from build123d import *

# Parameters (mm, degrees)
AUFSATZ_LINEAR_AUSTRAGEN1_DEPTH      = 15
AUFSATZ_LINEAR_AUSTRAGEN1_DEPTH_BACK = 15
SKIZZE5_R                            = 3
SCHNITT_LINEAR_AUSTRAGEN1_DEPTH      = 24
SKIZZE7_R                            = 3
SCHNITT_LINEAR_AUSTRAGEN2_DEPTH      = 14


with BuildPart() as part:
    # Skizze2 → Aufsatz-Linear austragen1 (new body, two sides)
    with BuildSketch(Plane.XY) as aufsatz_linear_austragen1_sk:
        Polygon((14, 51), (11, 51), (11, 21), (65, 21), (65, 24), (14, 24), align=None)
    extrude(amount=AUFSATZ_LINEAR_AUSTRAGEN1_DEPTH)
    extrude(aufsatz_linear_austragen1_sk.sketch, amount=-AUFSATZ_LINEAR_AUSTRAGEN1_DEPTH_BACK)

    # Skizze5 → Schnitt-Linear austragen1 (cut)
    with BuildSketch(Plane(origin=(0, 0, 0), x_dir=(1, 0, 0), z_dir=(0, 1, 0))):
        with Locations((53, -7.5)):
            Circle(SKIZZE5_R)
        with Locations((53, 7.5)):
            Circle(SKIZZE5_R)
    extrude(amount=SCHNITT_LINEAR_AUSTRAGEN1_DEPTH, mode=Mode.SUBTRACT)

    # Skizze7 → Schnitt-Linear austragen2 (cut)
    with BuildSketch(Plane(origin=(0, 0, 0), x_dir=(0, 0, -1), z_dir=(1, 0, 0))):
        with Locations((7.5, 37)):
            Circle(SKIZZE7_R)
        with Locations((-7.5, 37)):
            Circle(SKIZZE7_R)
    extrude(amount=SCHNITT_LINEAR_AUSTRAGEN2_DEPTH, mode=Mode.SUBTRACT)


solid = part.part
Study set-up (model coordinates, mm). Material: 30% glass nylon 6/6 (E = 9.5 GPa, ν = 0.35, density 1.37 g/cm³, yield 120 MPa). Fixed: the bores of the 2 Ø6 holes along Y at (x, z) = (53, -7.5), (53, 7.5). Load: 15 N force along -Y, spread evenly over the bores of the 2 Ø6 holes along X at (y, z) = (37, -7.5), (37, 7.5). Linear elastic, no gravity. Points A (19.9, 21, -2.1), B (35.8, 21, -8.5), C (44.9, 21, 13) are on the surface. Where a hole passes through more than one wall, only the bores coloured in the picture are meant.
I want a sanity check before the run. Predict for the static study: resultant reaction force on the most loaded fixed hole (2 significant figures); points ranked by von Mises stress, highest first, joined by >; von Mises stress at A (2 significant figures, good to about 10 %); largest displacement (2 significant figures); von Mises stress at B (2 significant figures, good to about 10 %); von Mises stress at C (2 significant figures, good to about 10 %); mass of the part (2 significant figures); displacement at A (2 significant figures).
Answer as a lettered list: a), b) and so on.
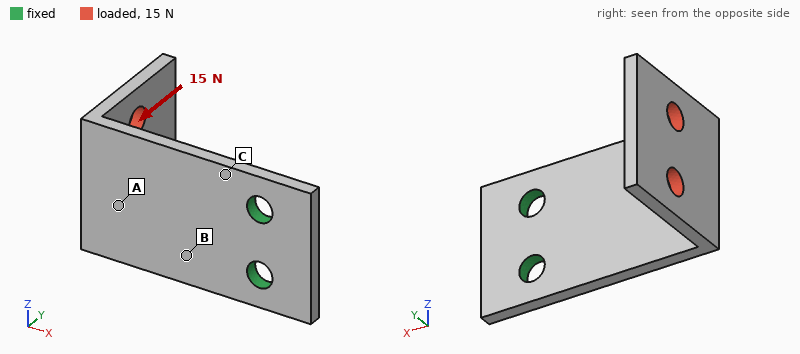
a) 7.5 N
b) C > B > A
c) 2.3 MPa
d) 0.65 mm
e) 7.3 MPa
f) 10 MPa
g) 9.5 g
h) 0.31 mm
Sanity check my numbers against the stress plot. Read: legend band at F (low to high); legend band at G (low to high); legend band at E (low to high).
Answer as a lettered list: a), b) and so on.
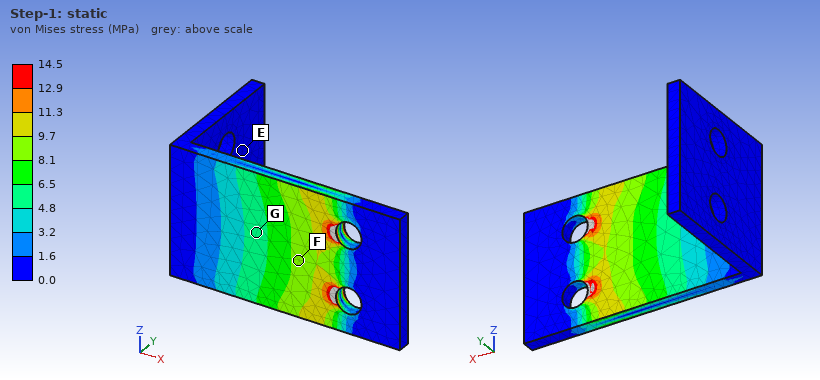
a) 8.1 to 9.7 MPa
b) 4.8 to 6.5 MPa
c) 0.0 to 1.6 MPa
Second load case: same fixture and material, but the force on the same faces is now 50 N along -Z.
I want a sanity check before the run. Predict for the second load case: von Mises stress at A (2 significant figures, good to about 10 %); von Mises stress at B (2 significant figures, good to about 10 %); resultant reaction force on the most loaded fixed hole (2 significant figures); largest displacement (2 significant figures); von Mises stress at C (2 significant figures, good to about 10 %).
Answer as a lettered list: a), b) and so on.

a) 10 MPa
b) 12 MPa
c) 110 N
d) 0.76 mm
e) 13 MPa
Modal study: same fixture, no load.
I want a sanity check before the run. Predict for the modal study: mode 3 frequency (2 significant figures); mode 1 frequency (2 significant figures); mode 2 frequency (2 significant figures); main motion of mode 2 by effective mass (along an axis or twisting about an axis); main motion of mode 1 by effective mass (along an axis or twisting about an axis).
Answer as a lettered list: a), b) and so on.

a) 1200 Hz
b) 390 Hz
c) 790 Hz
d) along Z
e) along Y
